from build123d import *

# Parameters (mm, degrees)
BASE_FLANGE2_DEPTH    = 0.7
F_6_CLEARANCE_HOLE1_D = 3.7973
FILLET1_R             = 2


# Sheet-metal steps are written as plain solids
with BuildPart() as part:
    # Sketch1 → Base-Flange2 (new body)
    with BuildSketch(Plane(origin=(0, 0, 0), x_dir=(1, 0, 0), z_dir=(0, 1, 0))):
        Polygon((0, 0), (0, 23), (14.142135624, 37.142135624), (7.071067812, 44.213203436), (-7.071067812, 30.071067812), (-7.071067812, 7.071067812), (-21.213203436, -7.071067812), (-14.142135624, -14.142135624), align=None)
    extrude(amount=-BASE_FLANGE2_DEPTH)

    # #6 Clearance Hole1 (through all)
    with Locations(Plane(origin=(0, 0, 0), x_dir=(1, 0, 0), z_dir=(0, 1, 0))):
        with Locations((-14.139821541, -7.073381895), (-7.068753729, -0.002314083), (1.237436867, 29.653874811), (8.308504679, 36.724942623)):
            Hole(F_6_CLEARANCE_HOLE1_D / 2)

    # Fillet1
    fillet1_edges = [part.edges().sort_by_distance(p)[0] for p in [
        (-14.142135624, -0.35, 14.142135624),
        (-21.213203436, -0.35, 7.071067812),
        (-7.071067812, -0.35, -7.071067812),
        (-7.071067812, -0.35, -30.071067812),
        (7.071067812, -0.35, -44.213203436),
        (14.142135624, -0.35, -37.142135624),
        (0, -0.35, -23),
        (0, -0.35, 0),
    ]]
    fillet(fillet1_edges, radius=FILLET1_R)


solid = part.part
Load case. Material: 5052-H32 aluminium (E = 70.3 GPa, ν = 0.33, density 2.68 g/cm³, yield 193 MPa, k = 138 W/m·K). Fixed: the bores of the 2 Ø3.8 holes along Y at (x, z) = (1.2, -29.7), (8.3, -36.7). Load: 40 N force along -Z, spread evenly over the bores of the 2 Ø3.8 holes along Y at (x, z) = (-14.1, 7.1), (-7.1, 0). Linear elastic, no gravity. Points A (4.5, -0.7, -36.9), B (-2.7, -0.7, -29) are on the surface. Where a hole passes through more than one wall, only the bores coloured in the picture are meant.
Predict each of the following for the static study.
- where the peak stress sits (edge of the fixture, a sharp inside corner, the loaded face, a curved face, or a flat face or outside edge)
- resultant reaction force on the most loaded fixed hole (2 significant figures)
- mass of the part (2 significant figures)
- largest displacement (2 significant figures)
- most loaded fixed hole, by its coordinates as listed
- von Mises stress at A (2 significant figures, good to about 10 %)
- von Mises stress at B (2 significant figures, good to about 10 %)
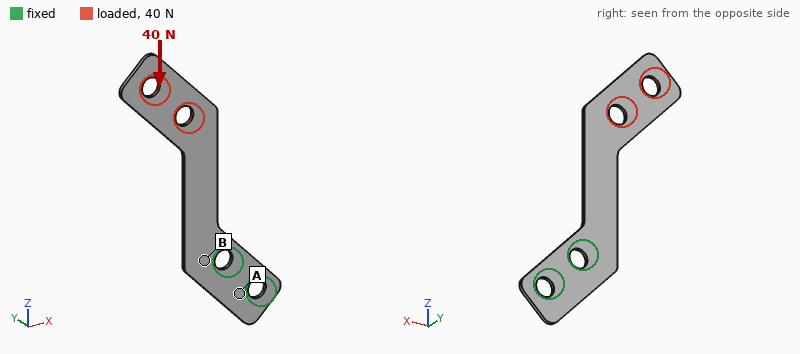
a curved face
47 N
0.96 g
0.17 mm
(1.2, -29.7)
8.3 MPa
25 MPa
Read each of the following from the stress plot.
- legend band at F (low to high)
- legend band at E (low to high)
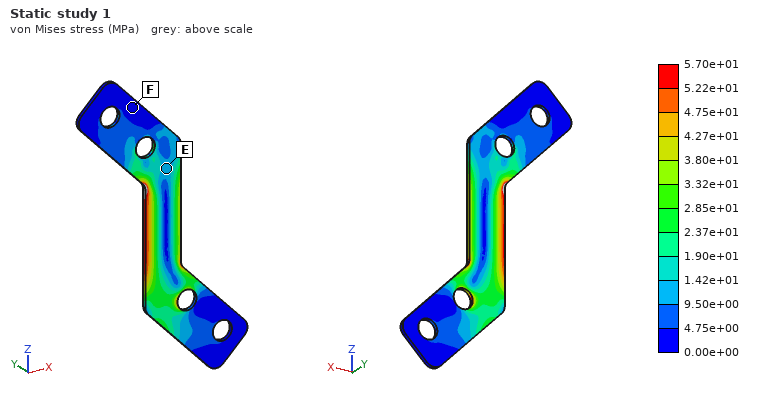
0.00e+00 to 4.75e+00 MPa
9.50e+00 to 1.42e+01 MPa
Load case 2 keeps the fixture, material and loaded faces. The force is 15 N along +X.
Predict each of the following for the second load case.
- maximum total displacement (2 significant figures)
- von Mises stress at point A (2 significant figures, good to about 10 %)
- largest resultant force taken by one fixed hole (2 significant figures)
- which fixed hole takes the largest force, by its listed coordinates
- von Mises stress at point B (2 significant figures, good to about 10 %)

0.18 mm
8.5 MPa
39 N
(1.2, -29.7)
25 MPa
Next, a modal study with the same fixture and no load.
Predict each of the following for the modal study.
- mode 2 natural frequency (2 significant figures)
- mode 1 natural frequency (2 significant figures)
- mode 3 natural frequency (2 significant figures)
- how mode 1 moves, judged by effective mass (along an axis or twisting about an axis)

1500 Hz
280 Hz
2600 Hz
along Y
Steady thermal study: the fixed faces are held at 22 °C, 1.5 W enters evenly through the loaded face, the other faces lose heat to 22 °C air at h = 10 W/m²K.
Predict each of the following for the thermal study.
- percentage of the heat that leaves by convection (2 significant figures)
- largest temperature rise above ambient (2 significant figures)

20 %
61 K
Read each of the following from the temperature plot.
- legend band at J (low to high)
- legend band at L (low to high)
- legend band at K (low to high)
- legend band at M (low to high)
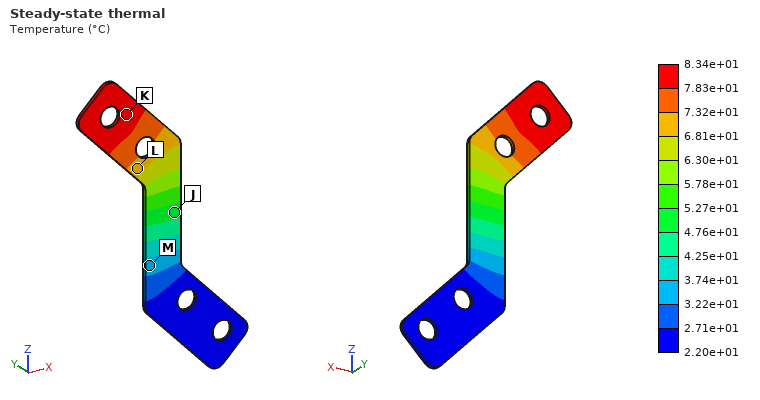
4.76e+01 to 5.27e+01 °C
6.81e+01 to 7.32e+01 °C
7.83e+01 to 8.34e+01 °C
3.22e+01 to 3.74e+01 °C
